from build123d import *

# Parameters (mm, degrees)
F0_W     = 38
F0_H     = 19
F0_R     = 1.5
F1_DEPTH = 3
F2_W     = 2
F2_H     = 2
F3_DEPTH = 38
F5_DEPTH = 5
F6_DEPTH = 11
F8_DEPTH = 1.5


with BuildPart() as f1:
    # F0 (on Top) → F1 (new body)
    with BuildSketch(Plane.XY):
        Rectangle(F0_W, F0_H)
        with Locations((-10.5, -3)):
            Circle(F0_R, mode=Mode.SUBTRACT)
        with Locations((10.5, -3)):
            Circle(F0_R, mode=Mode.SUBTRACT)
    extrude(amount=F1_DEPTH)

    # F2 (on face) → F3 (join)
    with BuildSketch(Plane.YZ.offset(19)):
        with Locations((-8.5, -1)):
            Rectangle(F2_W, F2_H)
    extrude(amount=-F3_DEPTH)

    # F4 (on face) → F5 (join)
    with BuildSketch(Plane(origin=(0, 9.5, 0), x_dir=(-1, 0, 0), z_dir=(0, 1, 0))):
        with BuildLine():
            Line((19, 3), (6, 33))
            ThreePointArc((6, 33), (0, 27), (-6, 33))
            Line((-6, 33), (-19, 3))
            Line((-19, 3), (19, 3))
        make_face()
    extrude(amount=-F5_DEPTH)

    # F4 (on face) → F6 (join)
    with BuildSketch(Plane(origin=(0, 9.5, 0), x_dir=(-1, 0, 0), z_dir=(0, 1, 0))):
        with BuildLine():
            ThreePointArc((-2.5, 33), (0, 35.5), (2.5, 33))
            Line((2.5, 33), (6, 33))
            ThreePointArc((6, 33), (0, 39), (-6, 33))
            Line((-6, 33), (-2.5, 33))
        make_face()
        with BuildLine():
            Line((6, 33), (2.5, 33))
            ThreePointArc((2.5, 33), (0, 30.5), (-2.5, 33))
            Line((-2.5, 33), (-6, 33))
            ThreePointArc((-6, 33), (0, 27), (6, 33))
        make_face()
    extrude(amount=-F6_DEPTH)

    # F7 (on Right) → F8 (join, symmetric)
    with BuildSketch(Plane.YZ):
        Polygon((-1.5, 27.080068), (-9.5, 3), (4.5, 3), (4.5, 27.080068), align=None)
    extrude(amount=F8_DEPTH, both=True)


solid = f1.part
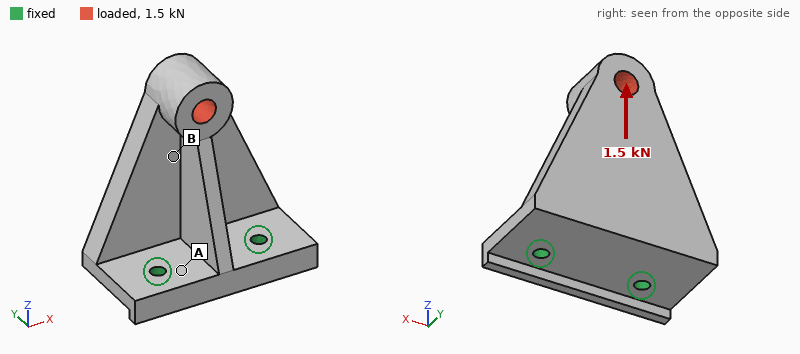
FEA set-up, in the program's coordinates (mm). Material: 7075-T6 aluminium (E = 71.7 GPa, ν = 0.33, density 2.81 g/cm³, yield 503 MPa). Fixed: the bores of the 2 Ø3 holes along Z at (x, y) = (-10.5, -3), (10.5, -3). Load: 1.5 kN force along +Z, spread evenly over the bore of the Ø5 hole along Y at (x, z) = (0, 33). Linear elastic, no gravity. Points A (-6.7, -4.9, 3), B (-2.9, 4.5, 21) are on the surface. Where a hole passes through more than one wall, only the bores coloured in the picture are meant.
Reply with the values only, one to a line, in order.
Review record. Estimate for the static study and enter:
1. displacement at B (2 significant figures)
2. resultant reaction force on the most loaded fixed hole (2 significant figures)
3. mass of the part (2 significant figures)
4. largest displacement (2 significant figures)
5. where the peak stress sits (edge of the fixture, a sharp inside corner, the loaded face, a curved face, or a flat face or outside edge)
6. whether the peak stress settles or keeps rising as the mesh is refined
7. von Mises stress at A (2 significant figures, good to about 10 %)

0.11 mm
750 N
21 g
0.18 mm
edge of the fixture
keeps rising
57 MPa
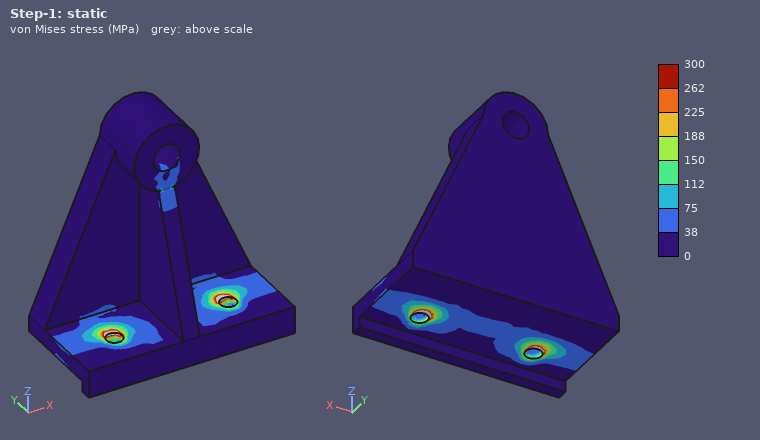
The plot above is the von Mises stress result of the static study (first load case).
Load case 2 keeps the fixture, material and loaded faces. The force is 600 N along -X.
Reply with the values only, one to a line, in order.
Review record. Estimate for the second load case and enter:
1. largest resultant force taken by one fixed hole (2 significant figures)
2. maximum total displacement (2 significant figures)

900 N
0.15 mm
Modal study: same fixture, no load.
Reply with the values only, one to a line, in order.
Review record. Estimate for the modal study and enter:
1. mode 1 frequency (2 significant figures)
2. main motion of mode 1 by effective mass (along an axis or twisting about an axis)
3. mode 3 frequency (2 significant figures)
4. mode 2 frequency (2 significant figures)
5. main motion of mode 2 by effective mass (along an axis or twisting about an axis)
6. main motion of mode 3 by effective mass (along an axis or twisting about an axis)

2500 Hz
along Y
11 kHz
4700 Hz
along X
along Z
